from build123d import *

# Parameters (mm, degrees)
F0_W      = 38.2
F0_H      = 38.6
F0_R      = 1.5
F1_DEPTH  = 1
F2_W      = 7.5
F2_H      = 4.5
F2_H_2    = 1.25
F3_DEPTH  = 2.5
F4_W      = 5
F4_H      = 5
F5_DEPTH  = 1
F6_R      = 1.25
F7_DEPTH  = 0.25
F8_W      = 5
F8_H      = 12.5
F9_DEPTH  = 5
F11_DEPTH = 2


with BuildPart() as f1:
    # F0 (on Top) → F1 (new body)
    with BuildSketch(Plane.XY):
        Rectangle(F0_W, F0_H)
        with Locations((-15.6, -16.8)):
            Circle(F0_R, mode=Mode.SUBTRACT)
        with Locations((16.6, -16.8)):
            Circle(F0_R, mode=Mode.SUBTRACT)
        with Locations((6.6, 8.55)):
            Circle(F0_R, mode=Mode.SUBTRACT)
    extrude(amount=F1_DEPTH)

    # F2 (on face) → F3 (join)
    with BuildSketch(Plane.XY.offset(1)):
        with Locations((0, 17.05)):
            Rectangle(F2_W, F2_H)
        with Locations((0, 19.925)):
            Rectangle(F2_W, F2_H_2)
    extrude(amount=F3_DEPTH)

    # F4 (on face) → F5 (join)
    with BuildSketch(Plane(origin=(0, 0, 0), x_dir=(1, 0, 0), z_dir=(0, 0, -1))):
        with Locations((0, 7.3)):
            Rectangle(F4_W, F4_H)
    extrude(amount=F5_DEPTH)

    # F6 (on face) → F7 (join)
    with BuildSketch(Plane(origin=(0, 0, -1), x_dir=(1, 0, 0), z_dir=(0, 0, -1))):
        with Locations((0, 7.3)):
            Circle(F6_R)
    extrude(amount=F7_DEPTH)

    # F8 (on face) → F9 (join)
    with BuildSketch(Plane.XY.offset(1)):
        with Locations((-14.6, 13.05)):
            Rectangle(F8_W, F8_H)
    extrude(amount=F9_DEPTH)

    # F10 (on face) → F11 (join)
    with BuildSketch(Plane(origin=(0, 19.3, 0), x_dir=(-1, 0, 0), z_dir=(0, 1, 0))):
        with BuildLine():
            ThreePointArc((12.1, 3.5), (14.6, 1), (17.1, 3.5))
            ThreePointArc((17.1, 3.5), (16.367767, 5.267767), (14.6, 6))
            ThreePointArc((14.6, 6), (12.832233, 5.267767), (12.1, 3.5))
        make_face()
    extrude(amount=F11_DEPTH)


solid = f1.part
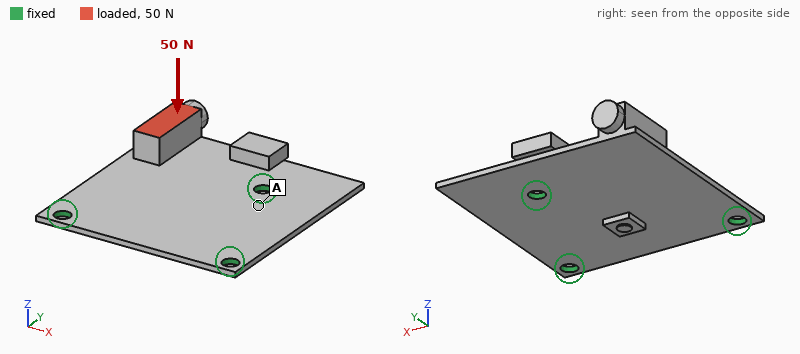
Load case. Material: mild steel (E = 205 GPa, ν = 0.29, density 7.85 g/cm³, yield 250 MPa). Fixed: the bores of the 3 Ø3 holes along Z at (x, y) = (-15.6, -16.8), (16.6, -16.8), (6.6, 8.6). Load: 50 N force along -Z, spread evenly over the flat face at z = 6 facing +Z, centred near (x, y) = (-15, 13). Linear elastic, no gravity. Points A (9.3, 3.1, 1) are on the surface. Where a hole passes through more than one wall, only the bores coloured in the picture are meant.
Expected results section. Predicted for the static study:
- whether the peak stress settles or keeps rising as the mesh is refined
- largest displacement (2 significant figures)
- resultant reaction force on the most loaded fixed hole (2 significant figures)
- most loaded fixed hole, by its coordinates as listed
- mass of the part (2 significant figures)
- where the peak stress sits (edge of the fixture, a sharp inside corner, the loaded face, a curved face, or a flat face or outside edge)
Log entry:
keeps rising
0.30 mm
44 N
(6.6, 8.6)
15 g
edge of the fixture
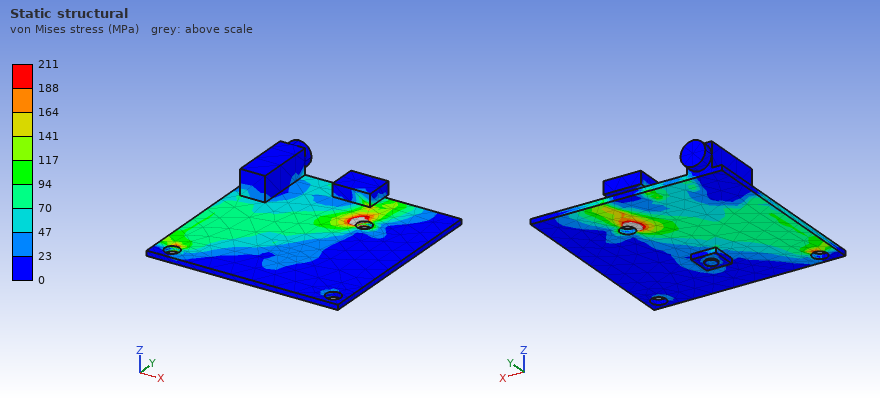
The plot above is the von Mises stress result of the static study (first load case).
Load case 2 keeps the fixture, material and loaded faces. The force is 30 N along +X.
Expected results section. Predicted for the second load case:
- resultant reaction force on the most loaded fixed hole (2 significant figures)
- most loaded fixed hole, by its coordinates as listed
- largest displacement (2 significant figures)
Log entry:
28 N
(6.6, 8.6)
60 µm
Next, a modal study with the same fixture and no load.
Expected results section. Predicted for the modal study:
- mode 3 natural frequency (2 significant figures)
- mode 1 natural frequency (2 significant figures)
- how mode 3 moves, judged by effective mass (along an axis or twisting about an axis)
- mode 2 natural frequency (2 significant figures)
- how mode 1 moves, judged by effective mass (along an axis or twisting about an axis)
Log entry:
5000 Hz
1100 Hz
along Z
3700 Hz
along Z
